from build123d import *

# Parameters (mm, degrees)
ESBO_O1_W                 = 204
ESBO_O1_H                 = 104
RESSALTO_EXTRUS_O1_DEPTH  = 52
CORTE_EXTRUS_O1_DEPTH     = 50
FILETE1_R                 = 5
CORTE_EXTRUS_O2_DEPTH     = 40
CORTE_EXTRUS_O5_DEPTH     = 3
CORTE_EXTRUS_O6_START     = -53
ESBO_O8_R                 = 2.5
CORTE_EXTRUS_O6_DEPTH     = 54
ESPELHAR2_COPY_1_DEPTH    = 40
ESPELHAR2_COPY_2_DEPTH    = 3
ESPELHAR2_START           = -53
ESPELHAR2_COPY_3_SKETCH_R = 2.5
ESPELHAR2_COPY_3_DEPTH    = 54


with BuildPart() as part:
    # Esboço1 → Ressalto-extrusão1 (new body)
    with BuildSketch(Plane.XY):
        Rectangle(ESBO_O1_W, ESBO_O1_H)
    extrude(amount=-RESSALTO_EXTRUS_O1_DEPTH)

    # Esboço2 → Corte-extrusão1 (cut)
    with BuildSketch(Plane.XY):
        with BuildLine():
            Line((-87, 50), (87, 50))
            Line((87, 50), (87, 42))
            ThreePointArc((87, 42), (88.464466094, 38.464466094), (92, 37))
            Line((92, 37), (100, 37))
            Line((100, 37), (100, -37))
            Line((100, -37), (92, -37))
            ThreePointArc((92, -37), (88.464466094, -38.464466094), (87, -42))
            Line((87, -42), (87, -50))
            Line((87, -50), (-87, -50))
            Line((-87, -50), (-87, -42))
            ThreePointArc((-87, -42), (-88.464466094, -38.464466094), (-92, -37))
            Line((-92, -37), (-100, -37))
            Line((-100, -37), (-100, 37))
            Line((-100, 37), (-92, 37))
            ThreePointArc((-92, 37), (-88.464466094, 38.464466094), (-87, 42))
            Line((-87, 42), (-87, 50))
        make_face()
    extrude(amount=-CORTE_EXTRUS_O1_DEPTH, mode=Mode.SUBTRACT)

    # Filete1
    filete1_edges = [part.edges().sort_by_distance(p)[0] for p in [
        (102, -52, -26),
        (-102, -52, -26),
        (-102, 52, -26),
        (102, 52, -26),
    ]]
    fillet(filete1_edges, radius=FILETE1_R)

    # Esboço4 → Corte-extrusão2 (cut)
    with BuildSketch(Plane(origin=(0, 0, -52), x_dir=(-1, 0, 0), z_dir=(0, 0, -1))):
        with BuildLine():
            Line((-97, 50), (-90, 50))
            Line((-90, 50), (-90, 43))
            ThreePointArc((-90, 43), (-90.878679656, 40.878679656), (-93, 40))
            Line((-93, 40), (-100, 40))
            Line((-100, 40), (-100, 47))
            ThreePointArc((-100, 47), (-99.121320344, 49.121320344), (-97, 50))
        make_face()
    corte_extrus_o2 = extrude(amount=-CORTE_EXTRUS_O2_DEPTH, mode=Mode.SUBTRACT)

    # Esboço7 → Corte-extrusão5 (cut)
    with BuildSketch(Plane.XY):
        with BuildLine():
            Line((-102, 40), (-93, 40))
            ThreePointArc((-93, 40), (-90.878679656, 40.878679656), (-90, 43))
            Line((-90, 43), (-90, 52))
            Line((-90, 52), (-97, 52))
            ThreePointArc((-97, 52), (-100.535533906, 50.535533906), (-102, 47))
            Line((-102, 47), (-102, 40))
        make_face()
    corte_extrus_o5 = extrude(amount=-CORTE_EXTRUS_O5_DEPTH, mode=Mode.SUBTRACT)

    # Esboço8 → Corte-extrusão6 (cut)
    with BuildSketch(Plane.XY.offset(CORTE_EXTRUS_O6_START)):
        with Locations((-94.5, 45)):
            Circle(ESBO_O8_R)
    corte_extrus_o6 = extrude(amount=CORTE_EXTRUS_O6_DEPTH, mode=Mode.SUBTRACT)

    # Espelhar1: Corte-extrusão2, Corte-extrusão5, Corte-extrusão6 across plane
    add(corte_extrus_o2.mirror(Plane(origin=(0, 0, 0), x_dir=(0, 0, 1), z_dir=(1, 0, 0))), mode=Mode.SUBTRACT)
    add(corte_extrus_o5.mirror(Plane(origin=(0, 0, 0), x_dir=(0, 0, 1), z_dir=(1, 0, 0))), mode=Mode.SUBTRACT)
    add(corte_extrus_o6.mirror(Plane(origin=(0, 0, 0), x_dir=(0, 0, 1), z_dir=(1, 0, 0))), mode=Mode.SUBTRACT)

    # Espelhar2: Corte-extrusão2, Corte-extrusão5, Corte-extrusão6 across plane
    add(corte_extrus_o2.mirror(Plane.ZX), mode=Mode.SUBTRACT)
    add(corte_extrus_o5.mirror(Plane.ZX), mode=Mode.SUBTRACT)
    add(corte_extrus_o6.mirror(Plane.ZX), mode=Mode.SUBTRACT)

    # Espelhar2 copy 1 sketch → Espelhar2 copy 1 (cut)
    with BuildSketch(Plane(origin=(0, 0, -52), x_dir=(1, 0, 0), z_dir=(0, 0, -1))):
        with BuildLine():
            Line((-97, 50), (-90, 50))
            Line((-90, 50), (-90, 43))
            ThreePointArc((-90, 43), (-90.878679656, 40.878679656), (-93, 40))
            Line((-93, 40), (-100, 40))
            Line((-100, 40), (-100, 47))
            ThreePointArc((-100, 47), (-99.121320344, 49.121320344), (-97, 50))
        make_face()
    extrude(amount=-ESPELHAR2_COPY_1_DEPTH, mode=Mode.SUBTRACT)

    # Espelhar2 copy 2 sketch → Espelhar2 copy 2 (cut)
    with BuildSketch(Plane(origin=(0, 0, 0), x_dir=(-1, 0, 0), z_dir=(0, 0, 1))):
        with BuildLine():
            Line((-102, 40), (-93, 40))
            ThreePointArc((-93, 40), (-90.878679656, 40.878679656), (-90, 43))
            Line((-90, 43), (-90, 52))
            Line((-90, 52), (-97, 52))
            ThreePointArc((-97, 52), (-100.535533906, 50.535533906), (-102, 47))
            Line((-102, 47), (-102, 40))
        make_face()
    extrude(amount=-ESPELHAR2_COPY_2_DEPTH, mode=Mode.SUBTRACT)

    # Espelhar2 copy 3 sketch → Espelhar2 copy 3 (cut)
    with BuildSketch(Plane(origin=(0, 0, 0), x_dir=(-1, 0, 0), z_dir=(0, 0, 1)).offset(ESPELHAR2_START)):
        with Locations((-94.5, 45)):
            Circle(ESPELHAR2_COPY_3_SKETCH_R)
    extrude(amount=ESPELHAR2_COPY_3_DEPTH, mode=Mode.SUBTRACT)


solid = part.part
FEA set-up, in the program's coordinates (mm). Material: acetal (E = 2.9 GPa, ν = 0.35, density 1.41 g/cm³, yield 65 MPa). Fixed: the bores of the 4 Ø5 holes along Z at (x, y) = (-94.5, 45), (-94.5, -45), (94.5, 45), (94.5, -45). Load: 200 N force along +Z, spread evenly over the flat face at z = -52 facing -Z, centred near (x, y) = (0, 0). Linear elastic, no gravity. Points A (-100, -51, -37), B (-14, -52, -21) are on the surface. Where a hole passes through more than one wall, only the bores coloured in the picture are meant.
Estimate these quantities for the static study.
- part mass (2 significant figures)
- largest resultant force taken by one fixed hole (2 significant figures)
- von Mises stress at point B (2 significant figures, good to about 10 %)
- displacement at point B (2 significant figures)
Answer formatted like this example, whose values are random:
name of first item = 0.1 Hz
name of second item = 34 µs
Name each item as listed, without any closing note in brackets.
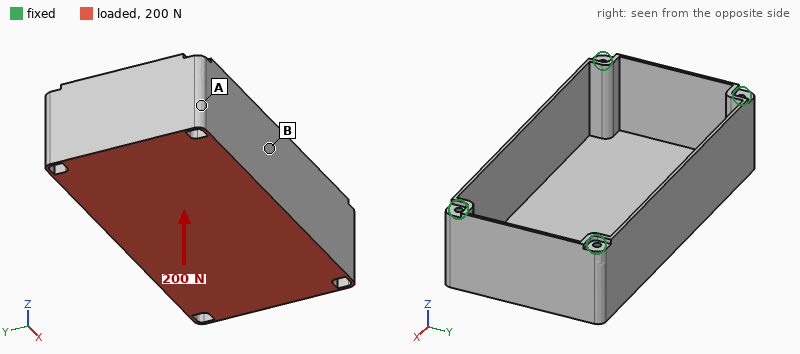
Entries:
part mass = 170 g
largest resultant force taken by one fixed hole = 59 N
von Mises stress at point B = 2.5 MPa
displacement at point B = 1.4 mm
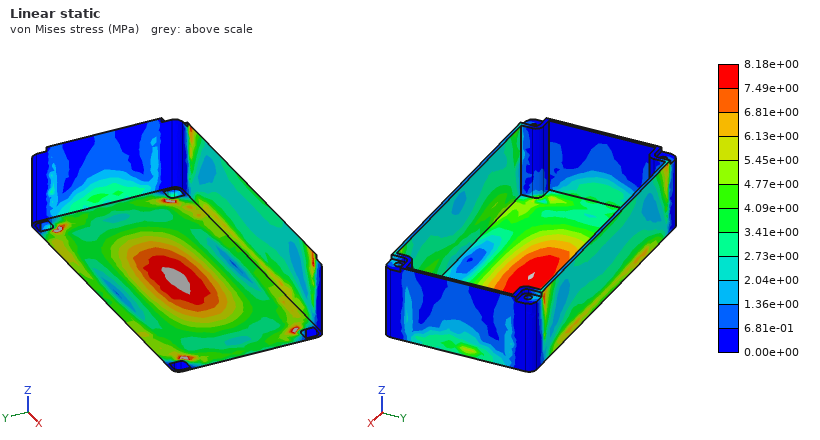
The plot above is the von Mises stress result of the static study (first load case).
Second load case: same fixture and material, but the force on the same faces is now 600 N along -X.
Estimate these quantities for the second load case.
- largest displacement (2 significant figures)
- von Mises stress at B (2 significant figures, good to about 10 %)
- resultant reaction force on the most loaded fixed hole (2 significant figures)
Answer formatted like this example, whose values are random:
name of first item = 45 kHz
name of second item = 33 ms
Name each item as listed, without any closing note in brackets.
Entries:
largest displacement = 89 µm
von Mises stress at B = 1.1 MPa
resultant reaction force on the most loaded fixed hole = 160 N
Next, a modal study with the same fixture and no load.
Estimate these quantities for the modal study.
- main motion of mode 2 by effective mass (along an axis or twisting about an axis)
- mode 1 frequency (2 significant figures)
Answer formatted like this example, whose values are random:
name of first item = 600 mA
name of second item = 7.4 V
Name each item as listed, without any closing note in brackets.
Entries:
main motion of mode 2 by effective mass = along Y
mode 1 frequency = 160 Hz
